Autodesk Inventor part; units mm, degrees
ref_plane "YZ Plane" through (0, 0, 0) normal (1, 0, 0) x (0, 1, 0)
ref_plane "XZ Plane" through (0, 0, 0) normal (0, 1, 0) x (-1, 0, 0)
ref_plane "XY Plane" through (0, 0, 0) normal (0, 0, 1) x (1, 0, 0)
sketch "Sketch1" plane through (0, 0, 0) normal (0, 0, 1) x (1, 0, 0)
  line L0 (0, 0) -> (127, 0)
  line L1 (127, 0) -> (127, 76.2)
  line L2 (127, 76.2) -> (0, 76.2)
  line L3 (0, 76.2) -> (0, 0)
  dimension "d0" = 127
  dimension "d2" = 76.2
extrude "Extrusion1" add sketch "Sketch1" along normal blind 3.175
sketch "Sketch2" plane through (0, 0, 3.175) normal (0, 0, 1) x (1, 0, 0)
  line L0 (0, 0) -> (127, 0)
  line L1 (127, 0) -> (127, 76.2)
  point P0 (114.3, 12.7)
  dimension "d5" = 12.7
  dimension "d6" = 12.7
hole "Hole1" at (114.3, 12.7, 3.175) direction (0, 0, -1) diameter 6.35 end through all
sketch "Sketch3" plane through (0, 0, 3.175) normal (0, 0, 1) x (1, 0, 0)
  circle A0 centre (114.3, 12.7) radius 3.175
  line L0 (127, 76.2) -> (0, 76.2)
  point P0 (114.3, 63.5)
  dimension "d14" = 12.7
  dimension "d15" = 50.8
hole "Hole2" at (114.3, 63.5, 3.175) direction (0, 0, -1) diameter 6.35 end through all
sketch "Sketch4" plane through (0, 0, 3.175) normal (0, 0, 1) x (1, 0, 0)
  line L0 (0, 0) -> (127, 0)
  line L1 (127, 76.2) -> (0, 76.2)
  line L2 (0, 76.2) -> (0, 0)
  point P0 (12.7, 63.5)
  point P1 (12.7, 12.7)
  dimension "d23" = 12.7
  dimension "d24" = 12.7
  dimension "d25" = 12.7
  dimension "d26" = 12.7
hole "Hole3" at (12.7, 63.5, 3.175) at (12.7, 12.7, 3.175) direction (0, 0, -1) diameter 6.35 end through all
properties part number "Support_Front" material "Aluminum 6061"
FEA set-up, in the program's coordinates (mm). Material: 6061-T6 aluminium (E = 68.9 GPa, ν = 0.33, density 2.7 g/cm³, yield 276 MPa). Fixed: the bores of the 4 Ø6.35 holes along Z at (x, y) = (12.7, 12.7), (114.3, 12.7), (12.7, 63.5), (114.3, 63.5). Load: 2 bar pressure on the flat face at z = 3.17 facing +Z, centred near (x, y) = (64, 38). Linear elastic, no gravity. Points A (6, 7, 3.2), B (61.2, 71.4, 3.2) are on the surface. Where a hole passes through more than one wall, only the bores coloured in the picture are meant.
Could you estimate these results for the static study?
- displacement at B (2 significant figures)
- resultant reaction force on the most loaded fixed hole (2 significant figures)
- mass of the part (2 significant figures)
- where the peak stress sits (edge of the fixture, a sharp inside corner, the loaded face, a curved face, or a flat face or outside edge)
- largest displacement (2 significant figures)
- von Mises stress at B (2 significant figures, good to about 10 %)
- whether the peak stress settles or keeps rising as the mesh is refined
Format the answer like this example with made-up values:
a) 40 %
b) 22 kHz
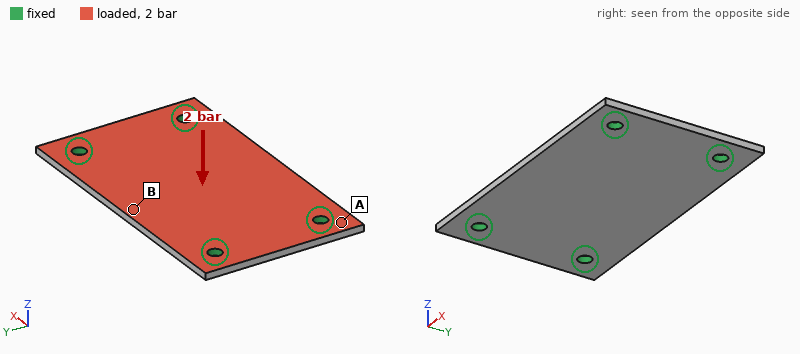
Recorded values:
a) 0.30 mm
b) 480 N
c) 82 g
d) edge of the fixture
e) 0.31 mm
f) 52 MPa
g) keeps rising
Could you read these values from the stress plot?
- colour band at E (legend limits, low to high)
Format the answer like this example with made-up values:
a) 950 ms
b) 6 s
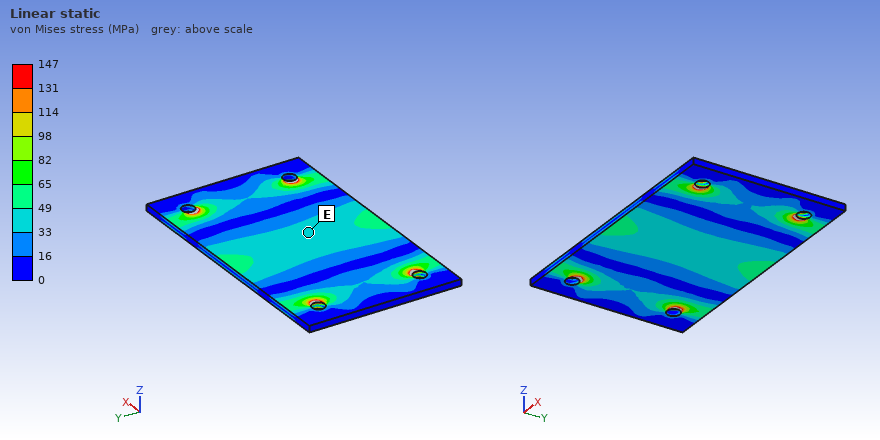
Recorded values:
a) 33 to 49 MPa
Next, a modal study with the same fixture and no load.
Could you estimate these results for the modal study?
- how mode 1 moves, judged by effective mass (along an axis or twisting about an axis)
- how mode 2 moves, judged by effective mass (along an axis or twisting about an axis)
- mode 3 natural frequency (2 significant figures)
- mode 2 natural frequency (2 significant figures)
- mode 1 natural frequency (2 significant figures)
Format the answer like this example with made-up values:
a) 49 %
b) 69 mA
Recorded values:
a) along Z
b) twisting about X
c) 4100 Hz
d) 2200 Hz
e) 1600 Hz
